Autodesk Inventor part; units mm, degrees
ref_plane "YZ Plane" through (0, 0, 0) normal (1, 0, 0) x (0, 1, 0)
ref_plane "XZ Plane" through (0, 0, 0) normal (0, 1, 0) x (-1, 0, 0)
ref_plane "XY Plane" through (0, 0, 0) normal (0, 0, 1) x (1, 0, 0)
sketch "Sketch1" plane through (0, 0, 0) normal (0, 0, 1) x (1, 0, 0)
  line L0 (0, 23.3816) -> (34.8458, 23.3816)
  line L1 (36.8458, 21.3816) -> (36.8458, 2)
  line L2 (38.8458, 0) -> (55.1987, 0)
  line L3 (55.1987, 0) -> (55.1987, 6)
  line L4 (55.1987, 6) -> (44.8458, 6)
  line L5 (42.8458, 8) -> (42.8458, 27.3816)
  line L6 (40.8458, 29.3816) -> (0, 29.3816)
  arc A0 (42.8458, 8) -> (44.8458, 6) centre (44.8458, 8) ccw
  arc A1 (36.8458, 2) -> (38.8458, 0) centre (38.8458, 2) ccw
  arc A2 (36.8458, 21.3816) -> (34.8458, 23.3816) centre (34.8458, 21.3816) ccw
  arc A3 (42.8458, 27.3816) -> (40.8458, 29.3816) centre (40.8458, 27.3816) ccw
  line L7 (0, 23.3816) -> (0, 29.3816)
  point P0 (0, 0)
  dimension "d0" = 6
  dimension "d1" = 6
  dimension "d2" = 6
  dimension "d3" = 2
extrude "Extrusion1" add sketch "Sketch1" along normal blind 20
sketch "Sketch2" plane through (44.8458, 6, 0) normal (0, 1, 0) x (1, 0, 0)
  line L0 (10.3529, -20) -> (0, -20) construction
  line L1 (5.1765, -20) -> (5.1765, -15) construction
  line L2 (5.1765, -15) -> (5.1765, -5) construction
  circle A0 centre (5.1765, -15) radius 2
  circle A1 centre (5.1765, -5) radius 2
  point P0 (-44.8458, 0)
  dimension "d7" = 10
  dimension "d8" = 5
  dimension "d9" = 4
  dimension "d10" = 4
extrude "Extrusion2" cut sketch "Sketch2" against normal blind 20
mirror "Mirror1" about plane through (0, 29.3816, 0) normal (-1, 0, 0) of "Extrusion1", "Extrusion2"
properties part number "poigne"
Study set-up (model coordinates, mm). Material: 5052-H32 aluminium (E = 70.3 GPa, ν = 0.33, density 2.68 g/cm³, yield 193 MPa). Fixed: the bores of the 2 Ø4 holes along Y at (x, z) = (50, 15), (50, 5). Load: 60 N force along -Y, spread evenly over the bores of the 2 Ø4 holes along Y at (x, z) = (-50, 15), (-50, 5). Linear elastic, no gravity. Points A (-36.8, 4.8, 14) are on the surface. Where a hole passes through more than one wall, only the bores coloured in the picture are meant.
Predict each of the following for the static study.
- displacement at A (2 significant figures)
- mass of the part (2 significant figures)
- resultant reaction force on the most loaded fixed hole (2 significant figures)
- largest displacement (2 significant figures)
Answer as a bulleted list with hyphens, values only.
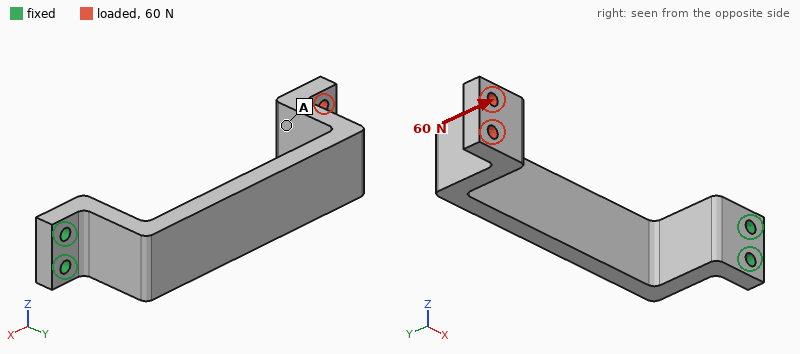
- 0.90 mm
- 50 g
- 61 N
- 1.2 mm
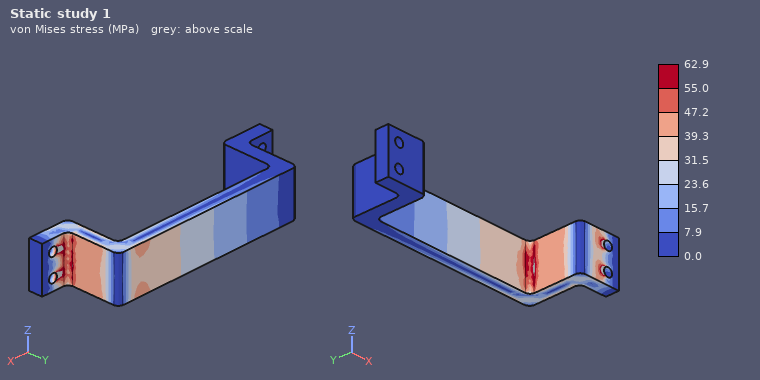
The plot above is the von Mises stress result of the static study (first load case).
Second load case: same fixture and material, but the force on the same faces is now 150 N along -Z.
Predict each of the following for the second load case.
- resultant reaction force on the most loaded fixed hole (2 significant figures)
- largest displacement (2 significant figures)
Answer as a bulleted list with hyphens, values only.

- 1.2 kN
- 1.1 mm
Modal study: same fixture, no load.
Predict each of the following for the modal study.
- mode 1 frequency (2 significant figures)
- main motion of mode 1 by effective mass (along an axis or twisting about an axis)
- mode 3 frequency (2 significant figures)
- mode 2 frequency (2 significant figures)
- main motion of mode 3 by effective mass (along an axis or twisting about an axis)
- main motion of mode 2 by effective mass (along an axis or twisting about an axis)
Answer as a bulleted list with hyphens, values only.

- 300 Hz
- along Y
- 1400 Hz
- 520 Hz
- along X
- along Z
